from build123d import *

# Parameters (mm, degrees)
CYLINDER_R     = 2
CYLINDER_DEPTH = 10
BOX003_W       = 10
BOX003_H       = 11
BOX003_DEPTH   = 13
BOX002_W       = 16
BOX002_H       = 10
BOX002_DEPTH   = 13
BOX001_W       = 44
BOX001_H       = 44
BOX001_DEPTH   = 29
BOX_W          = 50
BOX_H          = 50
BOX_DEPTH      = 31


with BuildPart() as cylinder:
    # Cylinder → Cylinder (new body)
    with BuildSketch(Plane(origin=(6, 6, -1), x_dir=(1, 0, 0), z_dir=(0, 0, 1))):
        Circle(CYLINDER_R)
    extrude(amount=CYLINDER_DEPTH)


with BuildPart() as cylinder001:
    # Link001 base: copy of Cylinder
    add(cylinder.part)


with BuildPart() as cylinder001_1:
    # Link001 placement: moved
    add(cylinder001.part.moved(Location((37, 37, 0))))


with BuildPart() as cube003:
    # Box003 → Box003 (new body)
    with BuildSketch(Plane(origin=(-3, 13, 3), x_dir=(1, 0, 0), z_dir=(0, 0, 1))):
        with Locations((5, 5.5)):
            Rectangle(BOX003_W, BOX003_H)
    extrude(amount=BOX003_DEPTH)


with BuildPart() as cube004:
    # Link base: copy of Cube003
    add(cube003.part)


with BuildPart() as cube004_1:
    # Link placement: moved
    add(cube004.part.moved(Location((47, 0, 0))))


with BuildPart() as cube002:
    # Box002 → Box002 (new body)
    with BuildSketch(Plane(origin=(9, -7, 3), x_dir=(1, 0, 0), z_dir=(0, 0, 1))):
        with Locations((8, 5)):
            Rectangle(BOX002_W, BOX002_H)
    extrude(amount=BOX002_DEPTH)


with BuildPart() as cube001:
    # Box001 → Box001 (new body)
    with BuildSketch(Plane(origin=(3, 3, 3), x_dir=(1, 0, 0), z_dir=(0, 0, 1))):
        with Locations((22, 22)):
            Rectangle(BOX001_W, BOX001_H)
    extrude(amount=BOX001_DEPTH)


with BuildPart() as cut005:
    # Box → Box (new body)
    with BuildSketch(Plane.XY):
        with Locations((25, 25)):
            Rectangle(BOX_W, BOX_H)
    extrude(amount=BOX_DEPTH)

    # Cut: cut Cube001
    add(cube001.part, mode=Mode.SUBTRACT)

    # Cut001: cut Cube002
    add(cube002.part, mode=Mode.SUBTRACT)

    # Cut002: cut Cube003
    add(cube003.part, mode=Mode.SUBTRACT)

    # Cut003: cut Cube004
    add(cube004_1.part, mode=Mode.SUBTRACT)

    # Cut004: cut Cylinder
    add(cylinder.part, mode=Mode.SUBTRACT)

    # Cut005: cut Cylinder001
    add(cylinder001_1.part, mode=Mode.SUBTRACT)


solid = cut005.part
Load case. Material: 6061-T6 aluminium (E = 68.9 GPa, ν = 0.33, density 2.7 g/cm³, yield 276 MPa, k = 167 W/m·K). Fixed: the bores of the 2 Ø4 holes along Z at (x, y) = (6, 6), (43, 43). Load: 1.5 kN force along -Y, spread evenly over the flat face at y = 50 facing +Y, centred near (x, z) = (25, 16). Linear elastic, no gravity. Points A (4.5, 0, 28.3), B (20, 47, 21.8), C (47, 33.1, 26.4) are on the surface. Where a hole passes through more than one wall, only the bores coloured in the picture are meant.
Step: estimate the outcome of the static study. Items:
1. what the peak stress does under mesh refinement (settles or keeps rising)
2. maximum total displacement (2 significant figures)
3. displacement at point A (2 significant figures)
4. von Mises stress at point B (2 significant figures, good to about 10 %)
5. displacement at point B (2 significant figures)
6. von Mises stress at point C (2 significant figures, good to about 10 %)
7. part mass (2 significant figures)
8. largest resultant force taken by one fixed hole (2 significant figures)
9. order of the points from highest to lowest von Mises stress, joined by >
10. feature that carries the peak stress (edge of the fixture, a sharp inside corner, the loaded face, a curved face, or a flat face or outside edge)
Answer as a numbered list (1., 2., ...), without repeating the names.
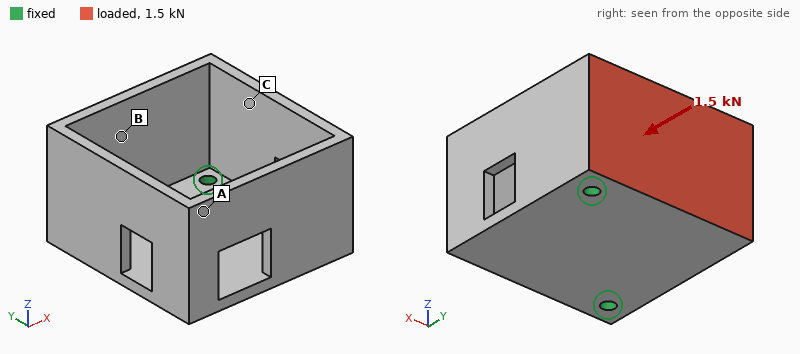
1. keeps rising
2. 0.25 mm
3. 0.11 mm
4. 44 MPa
5. 0.17 mm
6. 23 MPa
7. 59 g
8. 830 N
9. B > C > A
10. edge of the fixture
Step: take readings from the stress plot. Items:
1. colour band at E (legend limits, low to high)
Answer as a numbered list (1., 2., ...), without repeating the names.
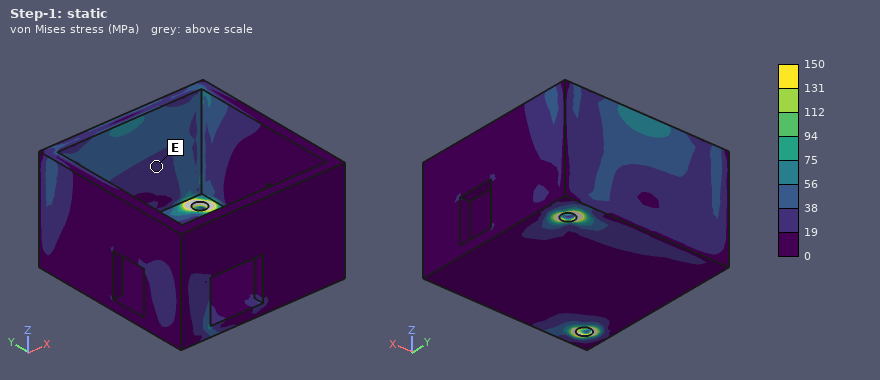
1. 19 to 38 MPa
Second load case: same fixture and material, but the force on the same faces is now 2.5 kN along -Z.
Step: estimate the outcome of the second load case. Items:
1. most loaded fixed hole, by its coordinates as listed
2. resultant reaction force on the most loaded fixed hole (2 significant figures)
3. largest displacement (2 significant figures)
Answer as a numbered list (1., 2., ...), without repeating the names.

1. (43, 43)
2. 2.1 kN
3. 0.78 mm
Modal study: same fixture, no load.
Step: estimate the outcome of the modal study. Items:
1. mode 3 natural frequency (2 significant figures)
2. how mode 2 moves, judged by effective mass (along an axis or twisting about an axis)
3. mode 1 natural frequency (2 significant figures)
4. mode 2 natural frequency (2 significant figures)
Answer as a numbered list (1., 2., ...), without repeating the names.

1. 5100 Hz
2. along Z
3. 1700 Hz
4. 2300 Hz
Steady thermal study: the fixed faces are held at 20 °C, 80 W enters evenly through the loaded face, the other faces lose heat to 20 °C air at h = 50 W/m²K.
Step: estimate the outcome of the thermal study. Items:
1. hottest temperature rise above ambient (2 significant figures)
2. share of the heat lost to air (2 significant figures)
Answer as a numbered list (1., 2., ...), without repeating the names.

1. 62 K
2. 21 %
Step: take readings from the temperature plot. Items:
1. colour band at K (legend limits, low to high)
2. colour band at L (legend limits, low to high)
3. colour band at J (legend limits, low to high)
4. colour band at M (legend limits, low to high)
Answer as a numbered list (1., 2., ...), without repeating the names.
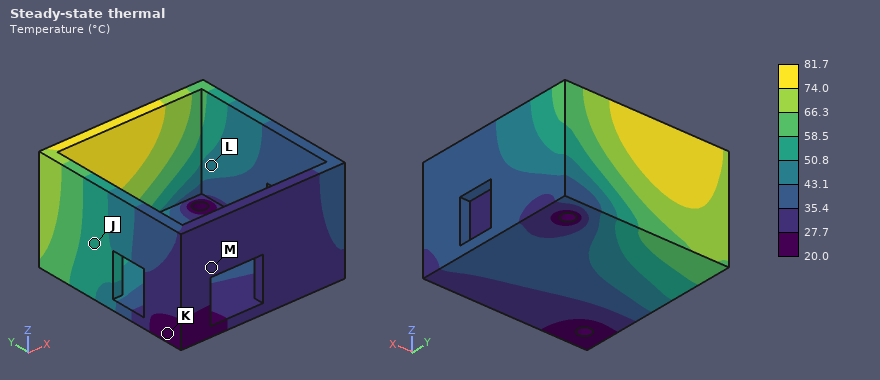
1. 20.0 to 27.7 °C
2. 43.1 to 50.8 °C
3. 50.8 to 58.5 °C
4. 27.7 to 35.4 °C
